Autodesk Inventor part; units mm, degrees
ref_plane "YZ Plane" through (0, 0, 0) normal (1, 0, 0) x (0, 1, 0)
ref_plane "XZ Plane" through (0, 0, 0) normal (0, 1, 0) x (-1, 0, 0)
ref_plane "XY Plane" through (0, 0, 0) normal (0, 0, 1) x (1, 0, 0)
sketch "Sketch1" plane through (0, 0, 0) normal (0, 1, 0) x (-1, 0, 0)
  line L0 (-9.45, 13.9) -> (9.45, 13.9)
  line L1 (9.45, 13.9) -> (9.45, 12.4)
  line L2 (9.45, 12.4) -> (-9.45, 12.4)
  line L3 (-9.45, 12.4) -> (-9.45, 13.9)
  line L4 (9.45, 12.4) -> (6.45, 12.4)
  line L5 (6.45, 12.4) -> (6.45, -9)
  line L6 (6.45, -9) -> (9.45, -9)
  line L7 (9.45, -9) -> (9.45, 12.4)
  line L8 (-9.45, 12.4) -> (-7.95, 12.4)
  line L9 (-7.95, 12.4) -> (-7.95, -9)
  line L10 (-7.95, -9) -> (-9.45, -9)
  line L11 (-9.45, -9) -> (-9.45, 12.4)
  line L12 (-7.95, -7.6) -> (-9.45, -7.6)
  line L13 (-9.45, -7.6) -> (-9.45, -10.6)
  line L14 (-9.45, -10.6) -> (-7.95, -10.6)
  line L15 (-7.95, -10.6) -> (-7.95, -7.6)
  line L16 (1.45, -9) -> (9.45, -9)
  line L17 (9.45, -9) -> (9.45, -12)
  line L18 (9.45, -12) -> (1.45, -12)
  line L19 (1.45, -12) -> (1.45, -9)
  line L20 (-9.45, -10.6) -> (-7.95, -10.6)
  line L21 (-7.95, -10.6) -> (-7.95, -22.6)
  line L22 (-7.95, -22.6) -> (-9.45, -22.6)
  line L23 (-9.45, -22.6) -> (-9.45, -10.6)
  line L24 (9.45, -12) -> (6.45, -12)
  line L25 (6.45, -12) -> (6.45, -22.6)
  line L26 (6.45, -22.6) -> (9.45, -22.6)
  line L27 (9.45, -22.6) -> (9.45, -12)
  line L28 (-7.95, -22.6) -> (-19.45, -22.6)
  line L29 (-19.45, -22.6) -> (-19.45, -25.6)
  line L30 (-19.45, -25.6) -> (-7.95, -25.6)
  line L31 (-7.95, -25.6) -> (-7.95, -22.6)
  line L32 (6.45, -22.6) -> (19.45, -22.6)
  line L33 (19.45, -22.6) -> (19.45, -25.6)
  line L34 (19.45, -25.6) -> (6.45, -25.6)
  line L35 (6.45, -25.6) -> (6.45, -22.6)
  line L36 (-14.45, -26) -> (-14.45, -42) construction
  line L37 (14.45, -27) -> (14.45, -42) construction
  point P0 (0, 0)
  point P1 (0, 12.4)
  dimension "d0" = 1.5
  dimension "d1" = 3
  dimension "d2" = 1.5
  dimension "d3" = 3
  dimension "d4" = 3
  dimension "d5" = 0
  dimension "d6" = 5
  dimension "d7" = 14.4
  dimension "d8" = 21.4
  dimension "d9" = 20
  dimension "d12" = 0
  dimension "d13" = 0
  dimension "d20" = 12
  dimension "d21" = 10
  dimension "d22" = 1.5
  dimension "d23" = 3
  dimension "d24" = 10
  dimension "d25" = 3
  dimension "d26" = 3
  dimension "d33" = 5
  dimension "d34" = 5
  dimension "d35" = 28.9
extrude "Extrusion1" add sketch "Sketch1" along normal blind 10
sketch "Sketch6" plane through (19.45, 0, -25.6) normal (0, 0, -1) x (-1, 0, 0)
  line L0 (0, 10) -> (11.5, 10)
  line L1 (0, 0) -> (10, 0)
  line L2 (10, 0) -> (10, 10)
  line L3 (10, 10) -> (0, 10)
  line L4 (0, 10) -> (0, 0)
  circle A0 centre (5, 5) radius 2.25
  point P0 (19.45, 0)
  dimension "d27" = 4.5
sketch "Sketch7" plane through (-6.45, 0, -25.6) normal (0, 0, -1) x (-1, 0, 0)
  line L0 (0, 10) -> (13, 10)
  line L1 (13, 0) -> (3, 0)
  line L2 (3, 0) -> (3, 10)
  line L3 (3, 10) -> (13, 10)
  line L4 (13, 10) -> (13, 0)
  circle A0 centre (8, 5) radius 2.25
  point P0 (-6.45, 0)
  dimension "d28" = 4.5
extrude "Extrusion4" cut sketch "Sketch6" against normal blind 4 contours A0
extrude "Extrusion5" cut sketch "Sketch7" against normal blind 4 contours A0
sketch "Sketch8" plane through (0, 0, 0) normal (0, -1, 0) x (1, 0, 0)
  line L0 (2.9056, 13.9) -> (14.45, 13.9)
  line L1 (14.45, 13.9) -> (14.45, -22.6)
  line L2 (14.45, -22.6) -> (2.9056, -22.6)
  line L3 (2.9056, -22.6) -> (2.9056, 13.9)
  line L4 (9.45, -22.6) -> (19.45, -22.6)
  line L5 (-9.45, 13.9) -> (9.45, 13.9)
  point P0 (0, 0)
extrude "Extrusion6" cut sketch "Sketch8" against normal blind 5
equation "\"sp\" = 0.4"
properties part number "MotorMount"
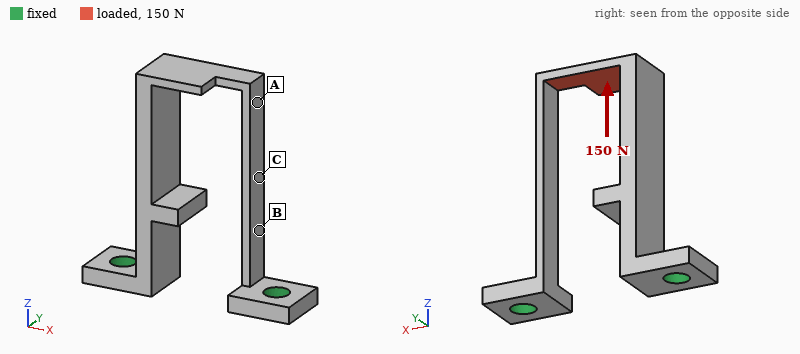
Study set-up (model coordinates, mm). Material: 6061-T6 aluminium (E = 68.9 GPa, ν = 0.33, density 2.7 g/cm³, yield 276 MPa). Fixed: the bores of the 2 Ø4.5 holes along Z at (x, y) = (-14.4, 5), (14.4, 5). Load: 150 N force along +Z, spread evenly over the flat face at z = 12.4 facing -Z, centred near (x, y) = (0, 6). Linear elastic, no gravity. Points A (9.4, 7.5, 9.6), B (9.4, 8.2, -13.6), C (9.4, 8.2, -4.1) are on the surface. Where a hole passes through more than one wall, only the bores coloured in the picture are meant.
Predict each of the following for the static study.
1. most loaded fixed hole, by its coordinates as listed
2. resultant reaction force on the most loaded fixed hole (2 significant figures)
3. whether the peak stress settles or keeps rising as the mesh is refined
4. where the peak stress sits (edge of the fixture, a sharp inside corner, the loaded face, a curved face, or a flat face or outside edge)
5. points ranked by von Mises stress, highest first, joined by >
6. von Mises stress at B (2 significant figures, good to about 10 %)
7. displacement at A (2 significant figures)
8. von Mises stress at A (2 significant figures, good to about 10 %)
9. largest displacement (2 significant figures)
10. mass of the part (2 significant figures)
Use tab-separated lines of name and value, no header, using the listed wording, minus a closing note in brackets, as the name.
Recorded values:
most loaded fixed hole, by its coordinates as listed	(-14.4, 5)
resultant reaction force on the most loaded fixed hole	90 N
whether the peak stress settles or keeps rising as the mesh is refined	keeps rising
where the peak stress sits	a sharp inside corner
points ranked by von Mises stress, highest first, joined by >	A > B > C
von Mises stress at B	22 MPa
displacement at A	0.11 mm
von Mises stress at A	38 MPa
largest displacement	0.11 mm
mass of the part	6.3 g
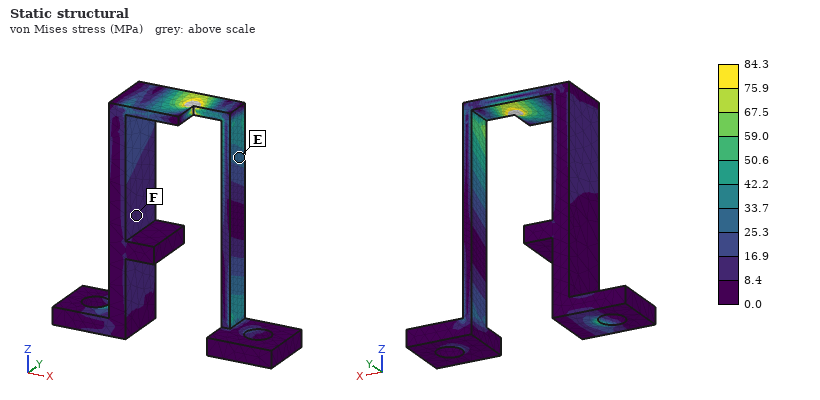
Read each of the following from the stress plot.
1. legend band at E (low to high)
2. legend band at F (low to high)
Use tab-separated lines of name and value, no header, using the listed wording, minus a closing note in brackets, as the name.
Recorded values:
legend band at E	25.3 to 33.7 MPa
legend band at F	8.4 to 16.9 MPa
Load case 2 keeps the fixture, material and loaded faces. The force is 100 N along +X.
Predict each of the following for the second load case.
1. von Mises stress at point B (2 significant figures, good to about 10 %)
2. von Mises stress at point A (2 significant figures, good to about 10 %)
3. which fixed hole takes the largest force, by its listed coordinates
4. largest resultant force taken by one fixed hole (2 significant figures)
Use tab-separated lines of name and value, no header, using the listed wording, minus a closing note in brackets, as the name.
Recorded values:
von Mises stress at point B	81 MPa
von Mises stress at point A	130 MPa
which fixed hole takes the largest force, by its listed coordinates	(-14.4, 5)
largest resultant force taken by one fixed hole	110 N
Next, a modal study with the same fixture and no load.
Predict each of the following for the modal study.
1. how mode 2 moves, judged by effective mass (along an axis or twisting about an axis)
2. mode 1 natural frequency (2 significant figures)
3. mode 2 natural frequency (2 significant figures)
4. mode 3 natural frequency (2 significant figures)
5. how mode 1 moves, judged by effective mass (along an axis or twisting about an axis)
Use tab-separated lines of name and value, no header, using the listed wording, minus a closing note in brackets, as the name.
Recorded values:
how mode 2 moves, judged by effective mass	along Y
mode 1 natural frequency	1500 Hz
mode 2 natural frequency	2300 Hz
mode 3 natural frequency	4600 Hz
how mode 1 moves, judged by effective mass	along X
